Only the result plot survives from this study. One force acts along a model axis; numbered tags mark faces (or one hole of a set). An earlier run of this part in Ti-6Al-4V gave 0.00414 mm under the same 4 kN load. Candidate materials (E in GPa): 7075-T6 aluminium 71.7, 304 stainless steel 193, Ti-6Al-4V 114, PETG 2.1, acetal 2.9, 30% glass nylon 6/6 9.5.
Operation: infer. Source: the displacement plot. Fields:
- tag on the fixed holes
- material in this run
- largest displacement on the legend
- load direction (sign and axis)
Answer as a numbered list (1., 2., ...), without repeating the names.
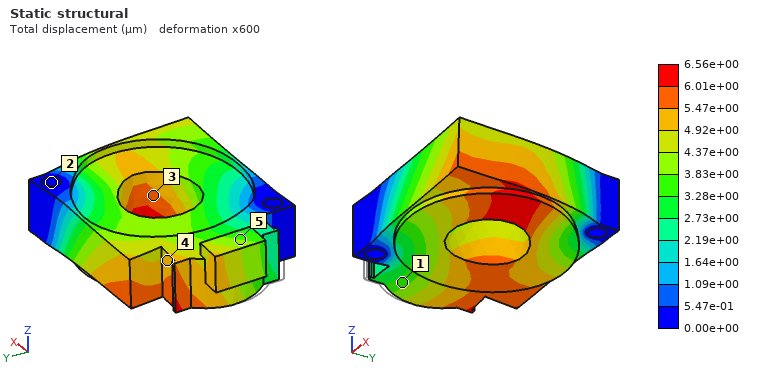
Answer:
1. 2
2. 7075-T6 aluminium
3. 6.56e+00 µm
4. +X
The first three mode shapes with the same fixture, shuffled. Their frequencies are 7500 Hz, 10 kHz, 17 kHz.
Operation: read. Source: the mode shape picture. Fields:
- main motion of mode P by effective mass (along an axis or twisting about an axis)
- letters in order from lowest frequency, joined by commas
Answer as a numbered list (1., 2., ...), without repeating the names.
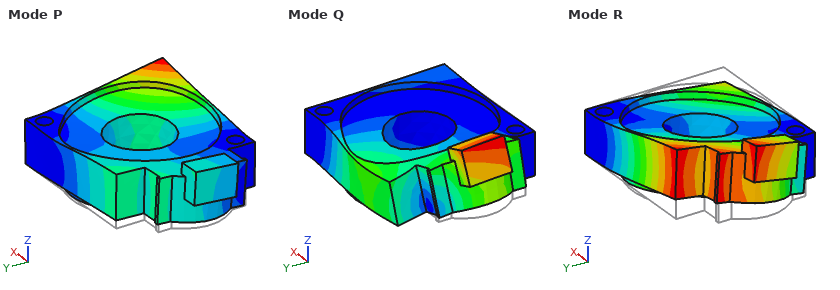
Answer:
1. along Z
2. R, P, Q
